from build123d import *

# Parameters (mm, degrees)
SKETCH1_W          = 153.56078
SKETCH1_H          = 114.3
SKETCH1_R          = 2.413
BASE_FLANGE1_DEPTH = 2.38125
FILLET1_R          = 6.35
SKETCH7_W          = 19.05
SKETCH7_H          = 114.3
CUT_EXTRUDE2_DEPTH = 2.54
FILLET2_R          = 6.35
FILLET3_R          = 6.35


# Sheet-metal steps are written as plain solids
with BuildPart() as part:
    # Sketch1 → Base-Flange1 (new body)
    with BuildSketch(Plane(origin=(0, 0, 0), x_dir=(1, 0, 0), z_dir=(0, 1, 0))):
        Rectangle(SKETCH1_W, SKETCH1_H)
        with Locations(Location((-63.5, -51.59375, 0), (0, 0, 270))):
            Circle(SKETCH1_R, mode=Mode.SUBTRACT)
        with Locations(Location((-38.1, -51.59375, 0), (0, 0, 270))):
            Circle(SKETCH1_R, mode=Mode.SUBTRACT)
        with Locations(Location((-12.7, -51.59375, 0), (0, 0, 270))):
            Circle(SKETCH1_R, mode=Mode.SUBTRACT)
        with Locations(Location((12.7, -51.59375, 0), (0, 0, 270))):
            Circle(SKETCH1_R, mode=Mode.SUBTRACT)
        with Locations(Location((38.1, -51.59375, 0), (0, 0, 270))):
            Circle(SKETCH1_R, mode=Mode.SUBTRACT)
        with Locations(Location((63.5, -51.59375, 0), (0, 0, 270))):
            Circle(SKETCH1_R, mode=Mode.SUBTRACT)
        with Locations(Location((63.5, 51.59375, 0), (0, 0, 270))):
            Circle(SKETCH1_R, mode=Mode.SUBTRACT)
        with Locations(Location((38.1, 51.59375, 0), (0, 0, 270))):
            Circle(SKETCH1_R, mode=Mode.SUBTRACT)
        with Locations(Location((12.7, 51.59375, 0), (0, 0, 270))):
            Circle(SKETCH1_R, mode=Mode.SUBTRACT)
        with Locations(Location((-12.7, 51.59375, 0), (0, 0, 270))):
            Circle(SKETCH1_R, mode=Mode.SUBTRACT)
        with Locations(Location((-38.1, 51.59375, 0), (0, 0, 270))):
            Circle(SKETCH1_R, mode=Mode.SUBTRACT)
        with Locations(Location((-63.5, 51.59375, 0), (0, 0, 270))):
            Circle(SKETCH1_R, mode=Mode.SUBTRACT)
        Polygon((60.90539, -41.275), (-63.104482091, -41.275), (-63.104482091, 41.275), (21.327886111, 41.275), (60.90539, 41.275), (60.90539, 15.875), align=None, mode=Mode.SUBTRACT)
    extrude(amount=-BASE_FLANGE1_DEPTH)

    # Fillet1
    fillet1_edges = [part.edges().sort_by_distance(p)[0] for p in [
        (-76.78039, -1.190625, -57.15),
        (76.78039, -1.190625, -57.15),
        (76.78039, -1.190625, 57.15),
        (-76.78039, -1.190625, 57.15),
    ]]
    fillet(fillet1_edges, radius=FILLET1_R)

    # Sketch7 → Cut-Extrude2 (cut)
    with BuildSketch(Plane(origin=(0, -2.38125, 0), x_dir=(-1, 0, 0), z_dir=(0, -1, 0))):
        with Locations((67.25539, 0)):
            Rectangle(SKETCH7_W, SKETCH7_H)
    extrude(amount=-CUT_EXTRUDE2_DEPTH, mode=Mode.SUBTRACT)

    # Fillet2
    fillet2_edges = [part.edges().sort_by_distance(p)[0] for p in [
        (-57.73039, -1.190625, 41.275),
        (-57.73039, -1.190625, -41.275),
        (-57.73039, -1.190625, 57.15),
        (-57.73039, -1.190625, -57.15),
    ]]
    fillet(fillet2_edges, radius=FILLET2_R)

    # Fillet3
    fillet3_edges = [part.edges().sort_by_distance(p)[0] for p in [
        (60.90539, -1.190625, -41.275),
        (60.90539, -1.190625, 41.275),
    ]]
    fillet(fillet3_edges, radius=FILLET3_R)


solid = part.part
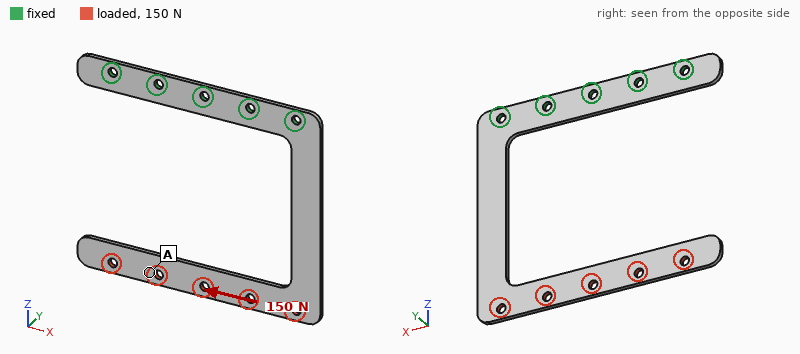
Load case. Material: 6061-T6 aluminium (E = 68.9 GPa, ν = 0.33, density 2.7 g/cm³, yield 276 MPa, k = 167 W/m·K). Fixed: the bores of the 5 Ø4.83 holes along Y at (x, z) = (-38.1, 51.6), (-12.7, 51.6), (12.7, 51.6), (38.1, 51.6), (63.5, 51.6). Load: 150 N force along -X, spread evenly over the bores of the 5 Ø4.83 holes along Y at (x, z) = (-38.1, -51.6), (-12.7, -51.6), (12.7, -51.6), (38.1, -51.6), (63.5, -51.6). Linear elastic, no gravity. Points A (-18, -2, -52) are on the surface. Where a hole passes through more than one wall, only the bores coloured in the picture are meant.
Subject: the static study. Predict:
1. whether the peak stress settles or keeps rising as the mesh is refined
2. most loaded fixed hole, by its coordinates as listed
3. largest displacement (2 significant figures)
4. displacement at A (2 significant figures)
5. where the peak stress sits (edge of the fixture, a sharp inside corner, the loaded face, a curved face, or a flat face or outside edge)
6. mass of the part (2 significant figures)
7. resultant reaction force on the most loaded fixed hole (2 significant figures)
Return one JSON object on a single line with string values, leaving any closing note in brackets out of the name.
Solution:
{"whether the peak stress settles or keeps rising as the mesh is refined": "keeps rising", "most loaded fixed hole, by its coordinates as listed": "(38.1, 51.6)", "largest displacement": "2.1 mm", "displacement at A": "1.6 mm", "where the peak stress sits": "edge of the fixture", "mass of the part": "34 g", "resultant reaction force on the most loaded fixed hole": "590 N"}
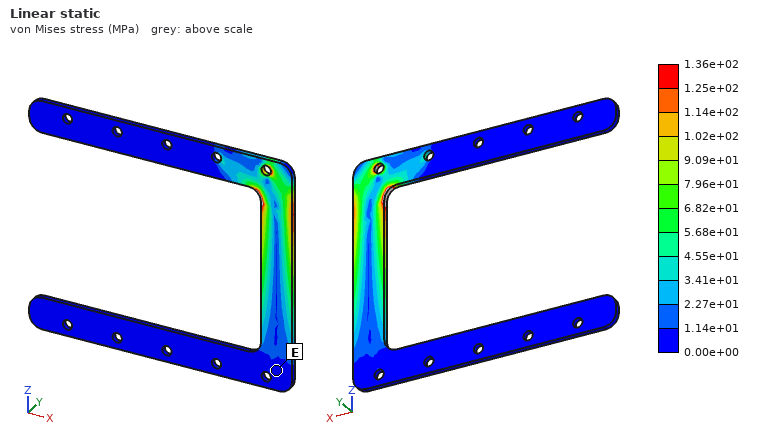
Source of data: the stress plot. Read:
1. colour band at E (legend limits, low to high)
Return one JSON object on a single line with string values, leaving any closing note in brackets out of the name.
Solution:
{"colour band at E": "0.00e+00 to 1.14e+01 MPa"}
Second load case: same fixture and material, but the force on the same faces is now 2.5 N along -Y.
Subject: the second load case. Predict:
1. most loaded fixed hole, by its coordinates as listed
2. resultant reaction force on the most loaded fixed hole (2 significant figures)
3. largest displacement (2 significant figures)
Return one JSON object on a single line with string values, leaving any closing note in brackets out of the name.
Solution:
{"most loaded fixed hole, by its coordinates as listed": "(63.5, 51.6)", "resultant reaction force on the most loaded fixed hole": "2.5 N", "largest displacement": "2.0 mm"}
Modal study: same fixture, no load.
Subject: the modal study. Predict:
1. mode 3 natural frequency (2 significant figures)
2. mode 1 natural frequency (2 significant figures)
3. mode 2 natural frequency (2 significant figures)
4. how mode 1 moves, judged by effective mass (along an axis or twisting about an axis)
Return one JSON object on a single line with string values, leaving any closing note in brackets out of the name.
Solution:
{"mode 3 natural frequency": "350 Hz", "mode 1 natural frequency": "58 Hz", "mode 2 natural frequency": "160 Hz", "how mode 1 moves, judged by effective mass": "along Y"}
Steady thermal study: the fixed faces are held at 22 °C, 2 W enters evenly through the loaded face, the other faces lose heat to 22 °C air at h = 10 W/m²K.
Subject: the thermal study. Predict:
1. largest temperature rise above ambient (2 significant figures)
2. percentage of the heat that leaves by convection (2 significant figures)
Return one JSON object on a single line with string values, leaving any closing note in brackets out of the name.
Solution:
{"largest temperature rise above ambient": "23 K", "percentage of the heat that leaves by convection": "57 %"}
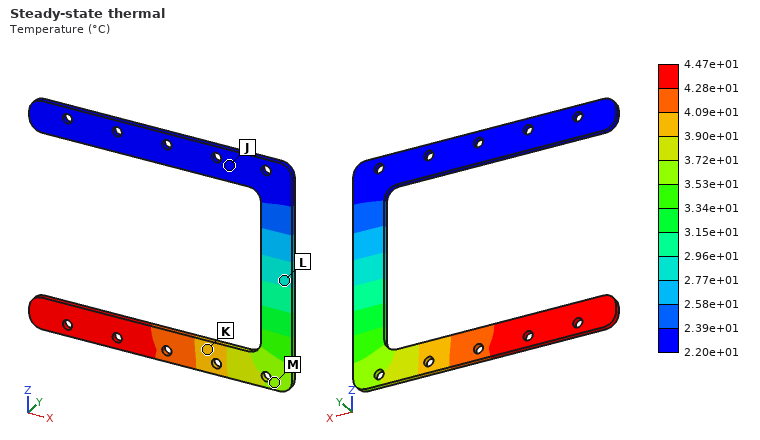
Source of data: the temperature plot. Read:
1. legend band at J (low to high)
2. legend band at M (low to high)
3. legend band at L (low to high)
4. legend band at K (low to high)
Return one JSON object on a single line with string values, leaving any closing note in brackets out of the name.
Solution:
{"legend band at J": "2.20e+01 to 2.39e+01 °C", "legend band at M": "3.53e+01 to 3.72e+01 °C", "legend band at L": "2.77e+01 to 2.96e+01 °C", "legend band at K": "3.90e+01 to 4.09e+01 °C"}
